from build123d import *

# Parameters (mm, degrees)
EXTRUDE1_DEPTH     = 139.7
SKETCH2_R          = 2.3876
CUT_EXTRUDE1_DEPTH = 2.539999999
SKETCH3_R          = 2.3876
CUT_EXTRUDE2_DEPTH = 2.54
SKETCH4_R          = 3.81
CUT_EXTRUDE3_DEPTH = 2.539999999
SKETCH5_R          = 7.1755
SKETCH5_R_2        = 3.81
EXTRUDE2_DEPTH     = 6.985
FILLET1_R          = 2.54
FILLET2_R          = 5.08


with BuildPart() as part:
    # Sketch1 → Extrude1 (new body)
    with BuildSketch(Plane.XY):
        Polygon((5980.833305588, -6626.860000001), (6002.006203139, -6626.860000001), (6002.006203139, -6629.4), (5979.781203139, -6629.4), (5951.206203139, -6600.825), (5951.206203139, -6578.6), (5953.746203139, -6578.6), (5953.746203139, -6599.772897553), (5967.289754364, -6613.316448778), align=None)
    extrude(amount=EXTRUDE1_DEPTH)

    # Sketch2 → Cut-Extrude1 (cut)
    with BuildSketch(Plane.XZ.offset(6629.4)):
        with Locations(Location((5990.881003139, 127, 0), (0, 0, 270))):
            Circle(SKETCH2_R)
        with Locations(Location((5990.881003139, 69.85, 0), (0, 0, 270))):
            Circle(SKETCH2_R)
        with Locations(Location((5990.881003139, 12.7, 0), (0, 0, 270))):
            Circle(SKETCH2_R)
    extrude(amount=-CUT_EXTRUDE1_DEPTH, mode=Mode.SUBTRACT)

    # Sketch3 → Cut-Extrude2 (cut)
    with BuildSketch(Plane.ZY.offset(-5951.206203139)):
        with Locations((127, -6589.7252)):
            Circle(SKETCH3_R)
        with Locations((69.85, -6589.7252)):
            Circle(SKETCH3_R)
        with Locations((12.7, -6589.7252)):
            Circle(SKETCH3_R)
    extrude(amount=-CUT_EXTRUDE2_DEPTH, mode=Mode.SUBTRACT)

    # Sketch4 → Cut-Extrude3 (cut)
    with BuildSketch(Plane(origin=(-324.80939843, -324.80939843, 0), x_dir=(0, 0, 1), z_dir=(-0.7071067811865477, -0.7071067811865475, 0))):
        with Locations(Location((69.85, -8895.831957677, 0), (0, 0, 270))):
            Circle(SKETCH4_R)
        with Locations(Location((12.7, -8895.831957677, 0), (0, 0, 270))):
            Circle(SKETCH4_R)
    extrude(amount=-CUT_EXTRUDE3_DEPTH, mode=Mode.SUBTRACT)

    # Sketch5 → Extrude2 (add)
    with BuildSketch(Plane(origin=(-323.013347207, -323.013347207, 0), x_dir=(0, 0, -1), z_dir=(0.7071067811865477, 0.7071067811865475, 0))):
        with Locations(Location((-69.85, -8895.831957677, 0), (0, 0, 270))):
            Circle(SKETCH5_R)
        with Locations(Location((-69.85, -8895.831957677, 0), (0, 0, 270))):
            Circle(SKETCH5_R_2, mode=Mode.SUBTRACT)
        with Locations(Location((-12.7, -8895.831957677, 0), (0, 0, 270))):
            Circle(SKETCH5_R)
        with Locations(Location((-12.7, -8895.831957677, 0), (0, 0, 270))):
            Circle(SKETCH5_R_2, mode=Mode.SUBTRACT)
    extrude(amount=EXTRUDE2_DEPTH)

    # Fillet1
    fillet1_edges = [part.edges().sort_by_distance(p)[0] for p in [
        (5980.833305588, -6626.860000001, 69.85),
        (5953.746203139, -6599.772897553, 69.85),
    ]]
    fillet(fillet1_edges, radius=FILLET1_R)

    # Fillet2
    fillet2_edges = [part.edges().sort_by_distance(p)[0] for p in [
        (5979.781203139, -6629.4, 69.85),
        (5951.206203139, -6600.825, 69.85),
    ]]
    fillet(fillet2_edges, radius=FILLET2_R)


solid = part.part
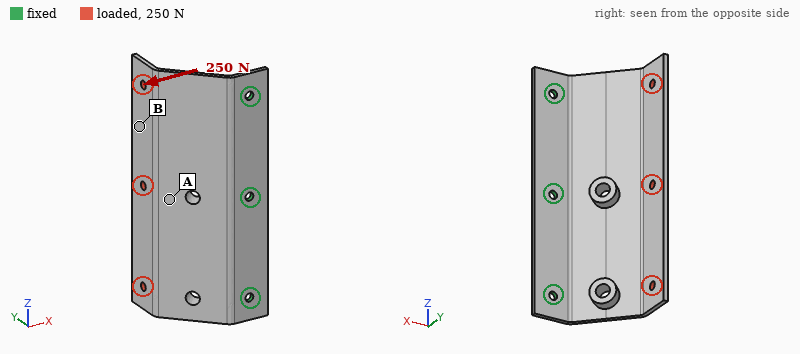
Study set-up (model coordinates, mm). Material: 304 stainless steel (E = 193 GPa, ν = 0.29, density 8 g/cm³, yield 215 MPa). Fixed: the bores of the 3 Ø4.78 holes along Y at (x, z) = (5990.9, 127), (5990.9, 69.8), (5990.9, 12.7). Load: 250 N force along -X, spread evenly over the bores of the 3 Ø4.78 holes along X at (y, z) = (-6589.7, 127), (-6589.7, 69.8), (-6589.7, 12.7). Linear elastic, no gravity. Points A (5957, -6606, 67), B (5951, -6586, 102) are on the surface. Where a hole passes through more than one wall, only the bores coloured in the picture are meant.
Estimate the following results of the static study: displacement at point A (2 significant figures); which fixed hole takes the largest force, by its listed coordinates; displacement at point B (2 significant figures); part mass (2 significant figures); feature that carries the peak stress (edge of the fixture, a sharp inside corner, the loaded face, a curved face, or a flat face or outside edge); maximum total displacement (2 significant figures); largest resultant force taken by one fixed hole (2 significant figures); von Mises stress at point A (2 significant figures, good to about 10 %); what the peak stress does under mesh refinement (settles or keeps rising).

0.22 mm
(5990.9, 69.8)
0.39 mm
240 g
edge of the fixture
0.47 mm
190 N
26 MPa
keeps rising
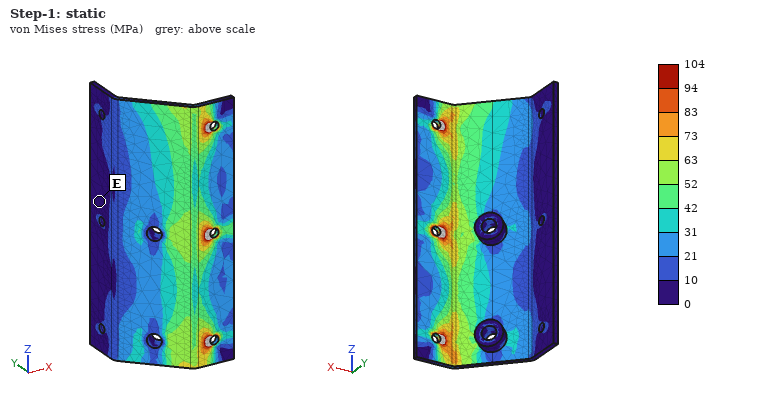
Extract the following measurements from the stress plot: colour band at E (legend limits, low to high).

0 to 10 MPa
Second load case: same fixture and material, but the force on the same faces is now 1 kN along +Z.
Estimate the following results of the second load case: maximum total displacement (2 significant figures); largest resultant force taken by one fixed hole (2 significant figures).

0.25 mm
550 N
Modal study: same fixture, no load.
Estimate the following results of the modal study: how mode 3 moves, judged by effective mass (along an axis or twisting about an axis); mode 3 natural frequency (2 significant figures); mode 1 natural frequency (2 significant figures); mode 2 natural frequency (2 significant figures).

along Y
2100 Hz
410 Hz
670 Hz
